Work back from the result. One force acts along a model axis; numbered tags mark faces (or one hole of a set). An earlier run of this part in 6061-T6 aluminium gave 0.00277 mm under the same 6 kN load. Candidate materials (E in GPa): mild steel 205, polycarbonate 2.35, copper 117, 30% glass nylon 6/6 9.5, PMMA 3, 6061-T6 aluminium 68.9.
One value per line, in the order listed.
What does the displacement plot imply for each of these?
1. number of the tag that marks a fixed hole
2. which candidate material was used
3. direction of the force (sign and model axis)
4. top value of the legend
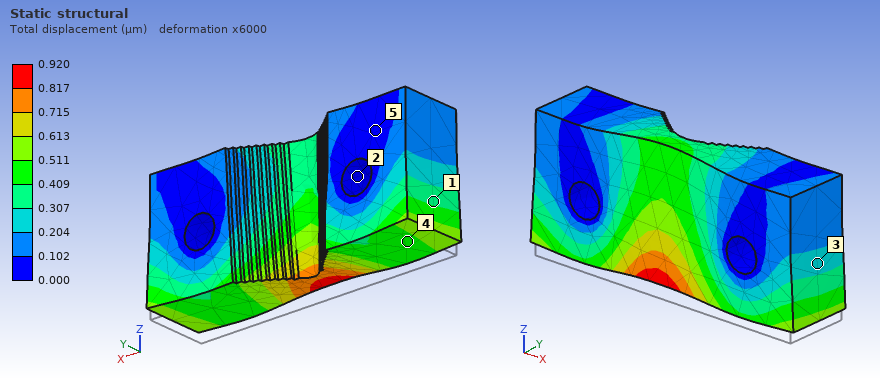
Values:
2
mild steel
+Z
0.920 µm
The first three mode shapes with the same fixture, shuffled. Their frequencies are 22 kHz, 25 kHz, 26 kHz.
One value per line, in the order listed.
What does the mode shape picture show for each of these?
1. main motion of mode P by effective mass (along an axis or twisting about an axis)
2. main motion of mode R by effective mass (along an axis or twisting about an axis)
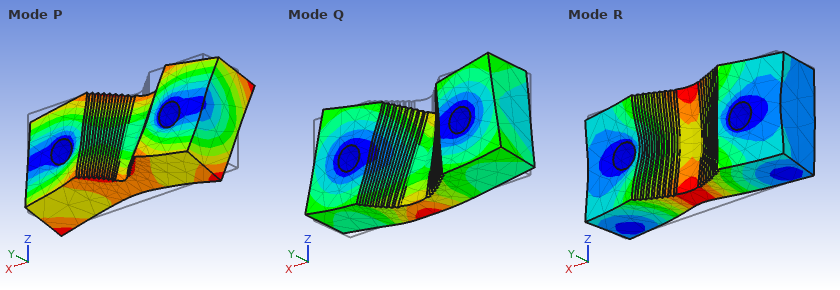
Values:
twisting about X
along Y
